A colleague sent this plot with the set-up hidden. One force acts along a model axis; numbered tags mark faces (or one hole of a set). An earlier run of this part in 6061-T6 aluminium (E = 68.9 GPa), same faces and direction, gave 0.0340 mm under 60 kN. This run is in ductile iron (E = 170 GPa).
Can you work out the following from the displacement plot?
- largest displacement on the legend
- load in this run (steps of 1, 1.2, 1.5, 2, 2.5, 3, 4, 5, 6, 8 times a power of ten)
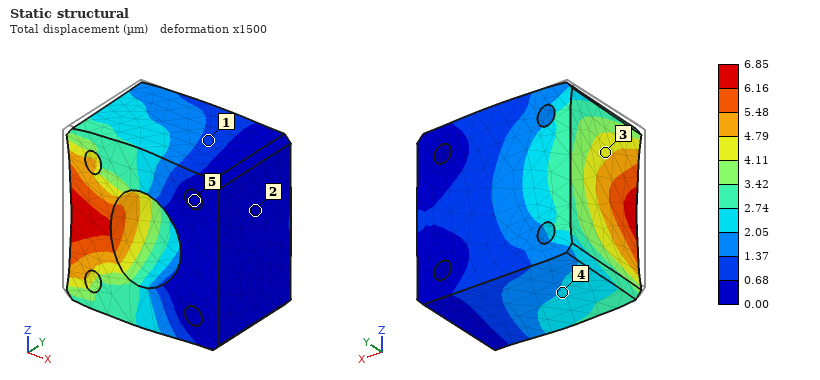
6.85 µm
30 kN
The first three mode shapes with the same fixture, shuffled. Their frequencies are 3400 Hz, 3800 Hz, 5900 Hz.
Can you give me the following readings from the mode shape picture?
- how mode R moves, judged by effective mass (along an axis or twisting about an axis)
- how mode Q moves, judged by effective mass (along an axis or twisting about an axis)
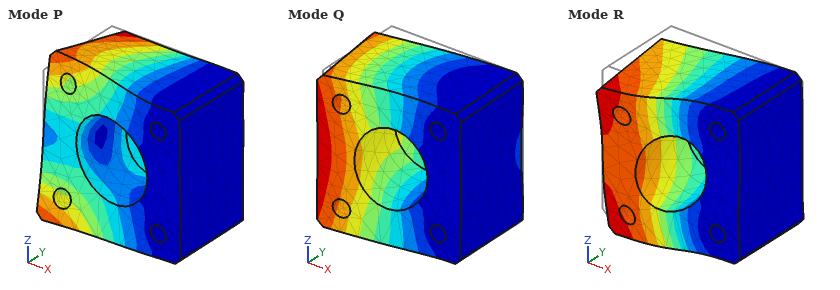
along Z
along Y
